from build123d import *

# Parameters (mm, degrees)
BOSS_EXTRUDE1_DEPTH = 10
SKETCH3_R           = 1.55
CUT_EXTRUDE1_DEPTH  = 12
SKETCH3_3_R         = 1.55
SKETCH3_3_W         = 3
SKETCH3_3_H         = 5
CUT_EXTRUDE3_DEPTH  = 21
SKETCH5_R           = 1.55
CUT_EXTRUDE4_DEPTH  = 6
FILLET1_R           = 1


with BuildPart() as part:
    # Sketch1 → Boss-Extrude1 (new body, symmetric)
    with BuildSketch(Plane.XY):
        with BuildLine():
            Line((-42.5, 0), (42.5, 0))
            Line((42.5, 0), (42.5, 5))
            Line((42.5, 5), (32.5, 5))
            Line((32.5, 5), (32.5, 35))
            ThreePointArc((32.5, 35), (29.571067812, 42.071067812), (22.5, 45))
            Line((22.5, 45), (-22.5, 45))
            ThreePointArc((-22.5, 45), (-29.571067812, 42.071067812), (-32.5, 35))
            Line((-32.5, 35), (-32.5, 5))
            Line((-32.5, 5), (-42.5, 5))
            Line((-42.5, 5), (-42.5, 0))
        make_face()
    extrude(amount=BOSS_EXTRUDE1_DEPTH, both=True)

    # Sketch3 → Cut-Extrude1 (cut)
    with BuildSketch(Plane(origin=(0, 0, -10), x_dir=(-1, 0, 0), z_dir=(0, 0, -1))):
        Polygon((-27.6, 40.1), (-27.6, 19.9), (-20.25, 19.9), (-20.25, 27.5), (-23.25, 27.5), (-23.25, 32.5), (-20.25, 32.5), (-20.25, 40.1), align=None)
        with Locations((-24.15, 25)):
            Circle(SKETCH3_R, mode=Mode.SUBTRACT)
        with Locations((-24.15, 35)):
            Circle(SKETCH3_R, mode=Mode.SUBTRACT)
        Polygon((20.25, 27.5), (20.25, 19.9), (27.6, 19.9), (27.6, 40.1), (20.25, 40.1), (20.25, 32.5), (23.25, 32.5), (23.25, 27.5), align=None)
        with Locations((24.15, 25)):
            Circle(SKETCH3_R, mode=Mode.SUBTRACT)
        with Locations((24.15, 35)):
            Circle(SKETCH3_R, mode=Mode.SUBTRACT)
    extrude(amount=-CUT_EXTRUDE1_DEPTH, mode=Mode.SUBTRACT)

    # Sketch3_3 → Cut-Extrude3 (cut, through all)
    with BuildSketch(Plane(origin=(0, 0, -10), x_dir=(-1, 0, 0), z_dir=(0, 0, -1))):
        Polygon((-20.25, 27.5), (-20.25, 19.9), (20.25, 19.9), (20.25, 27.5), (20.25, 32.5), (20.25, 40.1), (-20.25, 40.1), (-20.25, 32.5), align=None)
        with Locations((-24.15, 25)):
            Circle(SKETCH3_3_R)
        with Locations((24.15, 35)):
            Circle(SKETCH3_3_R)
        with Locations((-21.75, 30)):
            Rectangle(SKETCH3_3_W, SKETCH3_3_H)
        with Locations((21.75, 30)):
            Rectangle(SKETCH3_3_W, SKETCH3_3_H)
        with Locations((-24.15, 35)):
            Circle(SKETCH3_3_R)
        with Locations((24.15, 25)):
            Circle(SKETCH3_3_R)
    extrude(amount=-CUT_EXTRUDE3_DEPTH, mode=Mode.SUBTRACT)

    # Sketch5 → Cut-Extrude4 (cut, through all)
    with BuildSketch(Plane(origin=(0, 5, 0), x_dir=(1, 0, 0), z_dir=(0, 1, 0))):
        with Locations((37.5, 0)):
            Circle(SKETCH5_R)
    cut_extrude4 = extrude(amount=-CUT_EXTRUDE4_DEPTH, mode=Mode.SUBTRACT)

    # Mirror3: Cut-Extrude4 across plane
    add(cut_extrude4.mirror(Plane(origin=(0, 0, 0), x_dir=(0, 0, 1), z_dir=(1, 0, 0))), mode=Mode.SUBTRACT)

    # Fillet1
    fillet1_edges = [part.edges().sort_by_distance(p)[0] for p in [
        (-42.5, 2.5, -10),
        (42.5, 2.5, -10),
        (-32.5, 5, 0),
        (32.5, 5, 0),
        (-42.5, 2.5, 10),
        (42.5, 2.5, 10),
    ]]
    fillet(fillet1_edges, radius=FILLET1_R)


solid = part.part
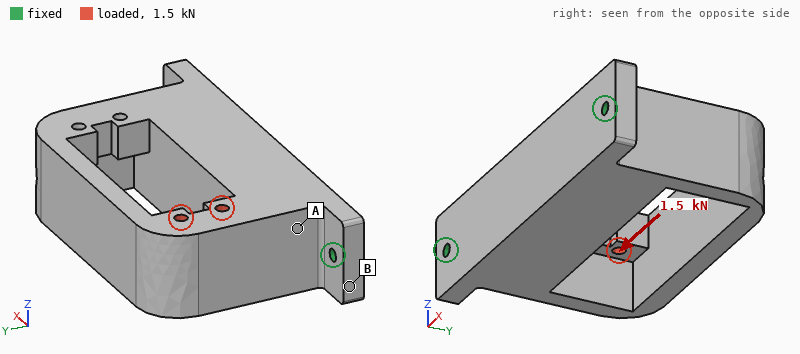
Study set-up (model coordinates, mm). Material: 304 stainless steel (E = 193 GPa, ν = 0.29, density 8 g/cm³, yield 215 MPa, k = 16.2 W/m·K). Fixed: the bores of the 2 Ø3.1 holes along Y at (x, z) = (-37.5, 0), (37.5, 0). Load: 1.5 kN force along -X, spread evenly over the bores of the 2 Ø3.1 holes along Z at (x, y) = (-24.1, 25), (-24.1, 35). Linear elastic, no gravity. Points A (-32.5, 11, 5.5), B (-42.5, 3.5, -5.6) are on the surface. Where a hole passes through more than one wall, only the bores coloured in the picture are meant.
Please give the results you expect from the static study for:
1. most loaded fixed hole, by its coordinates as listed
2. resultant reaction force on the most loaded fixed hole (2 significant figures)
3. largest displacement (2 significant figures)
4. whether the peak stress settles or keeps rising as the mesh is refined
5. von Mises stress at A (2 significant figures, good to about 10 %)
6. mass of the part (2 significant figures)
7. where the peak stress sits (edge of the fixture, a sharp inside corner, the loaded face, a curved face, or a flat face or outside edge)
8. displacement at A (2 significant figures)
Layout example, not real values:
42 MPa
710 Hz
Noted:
(37.5, 0)
1.1 kN
12 µm
keeps rising
18 MPa
310 g
edge of the fixture
2.2 µm
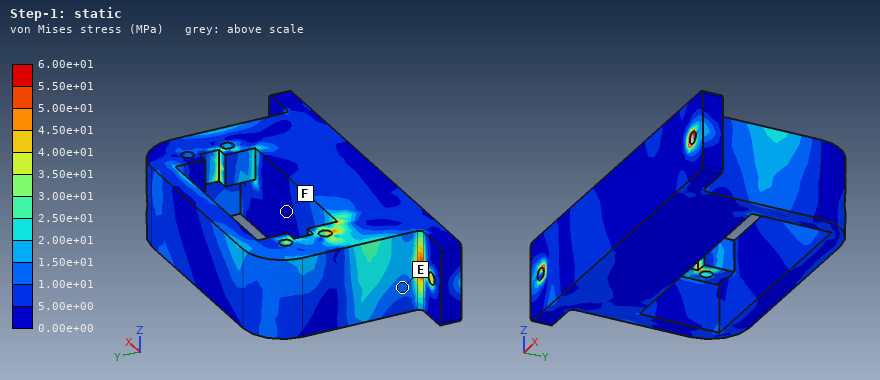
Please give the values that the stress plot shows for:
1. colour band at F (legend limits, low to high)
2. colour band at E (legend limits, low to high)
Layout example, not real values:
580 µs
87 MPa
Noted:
0.00e+00 to 5.00e+00 MPa
1.00e+01 to 1.50e+01 MPa
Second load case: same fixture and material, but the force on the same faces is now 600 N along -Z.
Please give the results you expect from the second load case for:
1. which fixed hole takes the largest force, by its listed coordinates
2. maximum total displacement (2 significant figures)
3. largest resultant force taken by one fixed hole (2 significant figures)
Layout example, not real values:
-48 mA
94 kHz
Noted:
(-37.5, 0)
56 µm
500 N
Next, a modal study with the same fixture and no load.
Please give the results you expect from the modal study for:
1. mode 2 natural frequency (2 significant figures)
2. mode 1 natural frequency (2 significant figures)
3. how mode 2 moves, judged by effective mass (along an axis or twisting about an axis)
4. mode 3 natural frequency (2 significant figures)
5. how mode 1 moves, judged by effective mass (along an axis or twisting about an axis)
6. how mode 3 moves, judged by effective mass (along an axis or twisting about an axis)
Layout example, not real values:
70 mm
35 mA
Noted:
5000 Hz
1600 Hz
along X
6200 Hz
along Z
along Y
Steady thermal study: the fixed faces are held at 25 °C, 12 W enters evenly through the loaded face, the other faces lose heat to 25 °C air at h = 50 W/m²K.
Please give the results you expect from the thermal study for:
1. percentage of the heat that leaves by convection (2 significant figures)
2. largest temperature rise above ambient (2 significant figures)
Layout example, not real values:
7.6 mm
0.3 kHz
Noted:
77 %
68 K
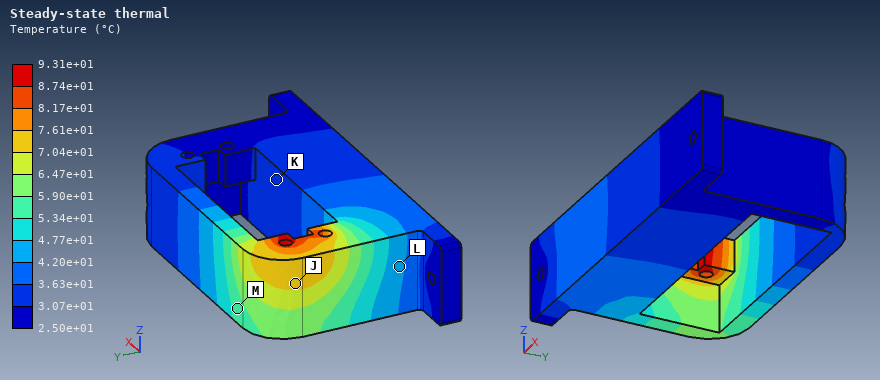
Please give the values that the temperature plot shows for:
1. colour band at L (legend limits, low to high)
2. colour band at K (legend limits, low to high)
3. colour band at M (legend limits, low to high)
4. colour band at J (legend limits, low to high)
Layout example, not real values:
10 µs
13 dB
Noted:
4.20e+01 to 4.77e+01 °C
3.07e+01 to 3.63e+01 °C
5.34e+01 to 5.90e+01 °C
7.04e+01 to 7.61e+01 °C
